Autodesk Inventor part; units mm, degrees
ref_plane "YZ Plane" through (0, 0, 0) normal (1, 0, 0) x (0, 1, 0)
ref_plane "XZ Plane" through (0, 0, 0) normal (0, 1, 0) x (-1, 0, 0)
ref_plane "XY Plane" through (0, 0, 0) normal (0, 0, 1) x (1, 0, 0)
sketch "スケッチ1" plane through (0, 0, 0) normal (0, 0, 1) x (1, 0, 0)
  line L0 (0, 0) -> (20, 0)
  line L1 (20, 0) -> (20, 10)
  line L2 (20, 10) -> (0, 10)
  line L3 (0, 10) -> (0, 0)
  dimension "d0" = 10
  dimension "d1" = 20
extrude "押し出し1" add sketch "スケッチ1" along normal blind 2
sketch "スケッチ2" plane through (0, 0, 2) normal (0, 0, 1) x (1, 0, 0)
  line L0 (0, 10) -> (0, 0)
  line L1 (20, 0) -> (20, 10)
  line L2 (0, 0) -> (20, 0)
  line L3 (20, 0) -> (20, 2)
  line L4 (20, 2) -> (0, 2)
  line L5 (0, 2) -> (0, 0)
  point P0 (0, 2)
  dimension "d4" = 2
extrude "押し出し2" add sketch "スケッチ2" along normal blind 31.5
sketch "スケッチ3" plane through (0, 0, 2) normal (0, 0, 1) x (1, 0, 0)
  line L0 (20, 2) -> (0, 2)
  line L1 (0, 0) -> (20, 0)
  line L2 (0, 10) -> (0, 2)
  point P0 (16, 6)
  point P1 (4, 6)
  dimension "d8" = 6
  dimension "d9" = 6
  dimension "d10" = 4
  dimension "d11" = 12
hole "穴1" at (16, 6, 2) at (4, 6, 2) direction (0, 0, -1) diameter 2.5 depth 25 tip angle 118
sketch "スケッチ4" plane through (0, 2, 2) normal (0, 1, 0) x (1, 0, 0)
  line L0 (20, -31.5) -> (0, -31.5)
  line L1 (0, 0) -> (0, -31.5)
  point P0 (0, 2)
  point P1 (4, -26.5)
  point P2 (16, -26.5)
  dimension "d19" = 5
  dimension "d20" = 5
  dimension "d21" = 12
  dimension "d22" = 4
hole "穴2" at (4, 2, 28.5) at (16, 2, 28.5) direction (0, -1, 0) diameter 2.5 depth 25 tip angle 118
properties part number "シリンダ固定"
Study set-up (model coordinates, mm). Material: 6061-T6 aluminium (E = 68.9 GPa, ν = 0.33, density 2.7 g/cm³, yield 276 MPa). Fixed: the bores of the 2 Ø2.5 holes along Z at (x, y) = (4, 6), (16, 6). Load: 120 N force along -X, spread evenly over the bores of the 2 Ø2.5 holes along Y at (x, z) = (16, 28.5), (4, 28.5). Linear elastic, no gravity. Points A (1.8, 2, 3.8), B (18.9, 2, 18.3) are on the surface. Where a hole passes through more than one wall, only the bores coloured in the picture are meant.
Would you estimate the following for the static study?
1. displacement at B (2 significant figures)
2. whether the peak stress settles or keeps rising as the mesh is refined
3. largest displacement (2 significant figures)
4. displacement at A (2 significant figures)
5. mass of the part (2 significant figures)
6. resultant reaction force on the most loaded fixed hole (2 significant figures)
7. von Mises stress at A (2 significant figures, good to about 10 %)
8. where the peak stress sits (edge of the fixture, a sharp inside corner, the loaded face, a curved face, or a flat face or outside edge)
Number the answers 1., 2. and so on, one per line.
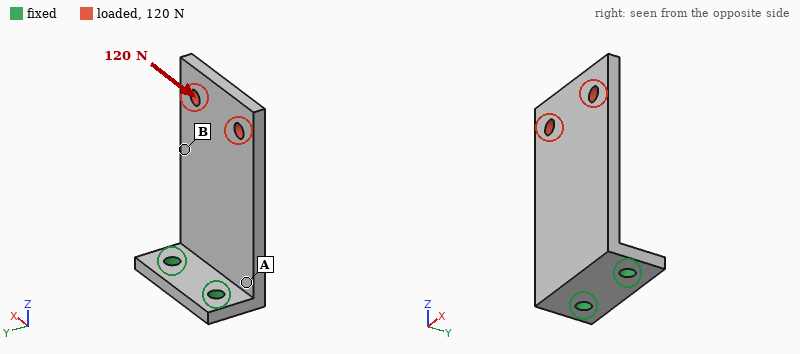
1. 53 µm
2. keeps rising
3. 91 µm
4. 19 µm
5. 4.4 g
6. 250 N
7. 54 MPa
8. edge of the fixture
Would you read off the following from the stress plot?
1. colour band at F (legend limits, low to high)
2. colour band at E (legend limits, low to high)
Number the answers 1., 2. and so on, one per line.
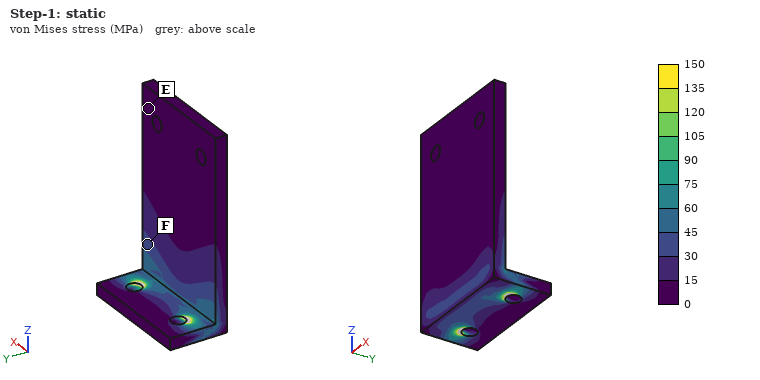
1. 30 to 45 MPa
2. 0 to 15 MPa
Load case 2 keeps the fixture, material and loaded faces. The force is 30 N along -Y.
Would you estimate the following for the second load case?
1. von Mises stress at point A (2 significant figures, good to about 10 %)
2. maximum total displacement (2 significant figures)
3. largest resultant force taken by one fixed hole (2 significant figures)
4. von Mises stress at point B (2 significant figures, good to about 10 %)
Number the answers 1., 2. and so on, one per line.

1. 48 MPa
2. 0.39 mm
3. 19 N
4. 23 MPa
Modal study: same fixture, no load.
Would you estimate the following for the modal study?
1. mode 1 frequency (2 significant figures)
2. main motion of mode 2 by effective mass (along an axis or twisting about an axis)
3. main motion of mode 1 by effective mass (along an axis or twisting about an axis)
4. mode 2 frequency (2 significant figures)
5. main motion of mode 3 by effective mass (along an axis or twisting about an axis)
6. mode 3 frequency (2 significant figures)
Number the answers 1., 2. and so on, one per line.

1. 1300 Hz
2. along X
3. along Y
4. 4600 Hz
5. along X
6. 5900 Hz
